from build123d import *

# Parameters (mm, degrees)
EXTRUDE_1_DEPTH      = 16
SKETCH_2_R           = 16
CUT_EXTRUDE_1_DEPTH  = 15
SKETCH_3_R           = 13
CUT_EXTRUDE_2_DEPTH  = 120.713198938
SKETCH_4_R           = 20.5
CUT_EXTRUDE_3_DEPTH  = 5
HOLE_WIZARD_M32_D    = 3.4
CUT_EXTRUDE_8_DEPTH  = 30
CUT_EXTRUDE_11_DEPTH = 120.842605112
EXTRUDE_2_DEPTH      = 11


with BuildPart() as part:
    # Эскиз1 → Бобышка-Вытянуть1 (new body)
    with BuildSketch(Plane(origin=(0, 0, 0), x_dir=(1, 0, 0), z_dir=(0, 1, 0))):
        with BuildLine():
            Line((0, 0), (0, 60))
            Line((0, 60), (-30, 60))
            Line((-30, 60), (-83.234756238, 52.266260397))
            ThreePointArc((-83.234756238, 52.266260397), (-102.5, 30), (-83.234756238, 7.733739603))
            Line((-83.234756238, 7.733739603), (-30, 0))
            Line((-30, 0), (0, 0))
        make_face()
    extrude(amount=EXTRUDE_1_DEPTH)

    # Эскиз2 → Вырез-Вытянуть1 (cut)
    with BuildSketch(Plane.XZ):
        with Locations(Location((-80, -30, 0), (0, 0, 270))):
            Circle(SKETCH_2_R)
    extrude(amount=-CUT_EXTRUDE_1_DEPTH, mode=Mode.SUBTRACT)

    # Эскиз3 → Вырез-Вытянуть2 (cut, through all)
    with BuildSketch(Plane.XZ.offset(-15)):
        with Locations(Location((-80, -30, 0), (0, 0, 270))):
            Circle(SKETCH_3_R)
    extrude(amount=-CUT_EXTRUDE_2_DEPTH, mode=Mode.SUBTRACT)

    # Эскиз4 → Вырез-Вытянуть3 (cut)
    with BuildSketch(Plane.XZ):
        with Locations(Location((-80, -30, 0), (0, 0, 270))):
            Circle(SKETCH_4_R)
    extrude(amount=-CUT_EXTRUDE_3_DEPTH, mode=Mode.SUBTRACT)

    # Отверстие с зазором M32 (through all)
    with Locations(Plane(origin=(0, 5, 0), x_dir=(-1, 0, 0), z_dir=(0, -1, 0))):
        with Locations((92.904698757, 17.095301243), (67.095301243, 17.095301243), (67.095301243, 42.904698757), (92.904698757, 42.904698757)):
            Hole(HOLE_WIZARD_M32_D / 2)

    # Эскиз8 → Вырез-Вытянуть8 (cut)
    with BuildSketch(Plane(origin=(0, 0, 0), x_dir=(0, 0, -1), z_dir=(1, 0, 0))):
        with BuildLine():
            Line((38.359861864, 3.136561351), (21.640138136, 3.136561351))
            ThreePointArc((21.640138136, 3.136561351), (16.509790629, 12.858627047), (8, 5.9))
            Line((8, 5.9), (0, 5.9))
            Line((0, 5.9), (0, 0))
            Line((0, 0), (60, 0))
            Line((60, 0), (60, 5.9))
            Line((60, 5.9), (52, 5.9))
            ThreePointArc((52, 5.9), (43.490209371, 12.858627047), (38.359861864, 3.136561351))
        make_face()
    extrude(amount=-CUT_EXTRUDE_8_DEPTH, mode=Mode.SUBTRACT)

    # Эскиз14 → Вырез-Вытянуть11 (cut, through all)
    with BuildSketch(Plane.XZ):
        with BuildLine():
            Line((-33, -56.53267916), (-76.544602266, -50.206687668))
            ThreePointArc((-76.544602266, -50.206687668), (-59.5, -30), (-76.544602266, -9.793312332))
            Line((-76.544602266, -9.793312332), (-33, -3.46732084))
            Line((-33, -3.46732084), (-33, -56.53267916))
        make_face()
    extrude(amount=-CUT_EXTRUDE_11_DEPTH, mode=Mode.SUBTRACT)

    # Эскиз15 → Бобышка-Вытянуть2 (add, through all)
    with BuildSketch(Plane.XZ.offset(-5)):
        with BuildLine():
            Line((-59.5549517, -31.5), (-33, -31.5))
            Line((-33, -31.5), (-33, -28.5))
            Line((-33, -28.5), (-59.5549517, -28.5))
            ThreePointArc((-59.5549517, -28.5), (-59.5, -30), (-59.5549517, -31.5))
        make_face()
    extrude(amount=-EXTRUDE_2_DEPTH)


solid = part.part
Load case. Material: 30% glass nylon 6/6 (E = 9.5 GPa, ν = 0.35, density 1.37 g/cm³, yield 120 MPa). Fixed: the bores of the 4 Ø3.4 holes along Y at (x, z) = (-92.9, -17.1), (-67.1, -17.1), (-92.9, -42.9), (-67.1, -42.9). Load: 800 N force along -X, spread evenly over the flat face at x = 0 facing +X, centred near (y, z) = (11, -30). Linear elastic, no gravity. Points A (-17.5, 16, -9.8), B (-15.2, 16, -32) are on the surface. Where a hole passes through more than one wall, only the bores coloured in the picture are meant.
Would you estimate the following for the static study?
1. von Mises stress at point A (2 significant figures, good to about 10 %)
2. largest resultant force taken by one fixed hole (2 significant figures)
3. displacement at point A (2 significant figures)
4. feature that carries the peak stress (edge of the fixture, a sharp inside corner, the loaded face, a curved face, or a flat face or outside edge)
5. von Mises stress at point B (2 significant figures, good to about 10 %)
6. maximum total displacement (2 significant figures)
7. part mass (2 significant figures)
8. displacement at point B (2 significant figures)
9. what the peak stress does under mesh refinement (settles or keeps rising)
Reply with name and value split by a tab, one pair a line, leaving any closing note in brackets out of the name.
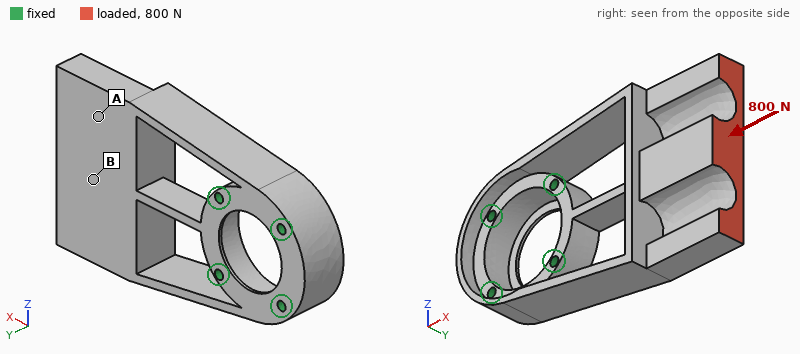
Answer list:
von Mises stress at point A	2.1 MPa
largest resultant force taken by one fixed hole	370 N
displacement at point A	0.13 mm
feature that carries the peak stress	edge of the fixture
von Mises stress at point B	1.3 MPa
maximum total displacement	0.19 mm
part mass	42 g
displacement at point B	0.14 mm
what the peak stress does under mesh refinement	keeps rising
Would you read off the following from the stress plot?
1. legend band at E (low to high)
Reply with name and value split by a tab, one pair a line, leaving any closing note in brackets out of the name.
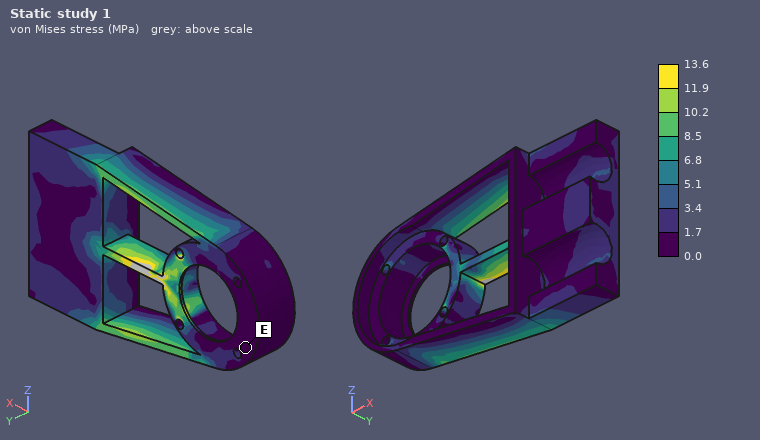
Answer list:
legend band at E	0.0 to 1.7 MPa
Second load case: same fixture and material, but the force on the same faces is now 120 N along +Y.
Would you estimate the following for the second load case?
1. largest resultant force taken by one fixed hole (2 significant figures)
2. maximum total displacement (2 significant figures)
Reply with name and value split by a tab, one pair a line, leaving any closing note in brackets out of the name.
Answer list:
largest resultant force taken by one fixed hole	170 N
maximum total displacement	1.0 mm
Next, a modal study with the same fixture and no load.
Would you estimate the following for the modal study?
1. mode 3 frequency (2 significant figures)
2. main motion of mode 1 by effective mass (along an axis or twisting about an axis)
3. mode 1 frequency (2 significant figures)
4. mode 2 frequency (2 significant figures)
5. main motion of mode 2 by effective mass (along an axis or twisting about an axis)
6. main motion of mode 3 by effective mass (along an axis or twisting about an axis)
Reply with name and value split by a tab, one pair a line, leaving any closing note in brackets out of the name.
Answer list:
mode 3 frequency	980 Hz
main motion of mode 1 by effective mass	along Z
mode 1 frequency	370 Hz
mode 2 frequency	490 Hz
main motion of mode 2 by effective mass	along Y
main motion of mode 3 by effective mass	twisting about X
